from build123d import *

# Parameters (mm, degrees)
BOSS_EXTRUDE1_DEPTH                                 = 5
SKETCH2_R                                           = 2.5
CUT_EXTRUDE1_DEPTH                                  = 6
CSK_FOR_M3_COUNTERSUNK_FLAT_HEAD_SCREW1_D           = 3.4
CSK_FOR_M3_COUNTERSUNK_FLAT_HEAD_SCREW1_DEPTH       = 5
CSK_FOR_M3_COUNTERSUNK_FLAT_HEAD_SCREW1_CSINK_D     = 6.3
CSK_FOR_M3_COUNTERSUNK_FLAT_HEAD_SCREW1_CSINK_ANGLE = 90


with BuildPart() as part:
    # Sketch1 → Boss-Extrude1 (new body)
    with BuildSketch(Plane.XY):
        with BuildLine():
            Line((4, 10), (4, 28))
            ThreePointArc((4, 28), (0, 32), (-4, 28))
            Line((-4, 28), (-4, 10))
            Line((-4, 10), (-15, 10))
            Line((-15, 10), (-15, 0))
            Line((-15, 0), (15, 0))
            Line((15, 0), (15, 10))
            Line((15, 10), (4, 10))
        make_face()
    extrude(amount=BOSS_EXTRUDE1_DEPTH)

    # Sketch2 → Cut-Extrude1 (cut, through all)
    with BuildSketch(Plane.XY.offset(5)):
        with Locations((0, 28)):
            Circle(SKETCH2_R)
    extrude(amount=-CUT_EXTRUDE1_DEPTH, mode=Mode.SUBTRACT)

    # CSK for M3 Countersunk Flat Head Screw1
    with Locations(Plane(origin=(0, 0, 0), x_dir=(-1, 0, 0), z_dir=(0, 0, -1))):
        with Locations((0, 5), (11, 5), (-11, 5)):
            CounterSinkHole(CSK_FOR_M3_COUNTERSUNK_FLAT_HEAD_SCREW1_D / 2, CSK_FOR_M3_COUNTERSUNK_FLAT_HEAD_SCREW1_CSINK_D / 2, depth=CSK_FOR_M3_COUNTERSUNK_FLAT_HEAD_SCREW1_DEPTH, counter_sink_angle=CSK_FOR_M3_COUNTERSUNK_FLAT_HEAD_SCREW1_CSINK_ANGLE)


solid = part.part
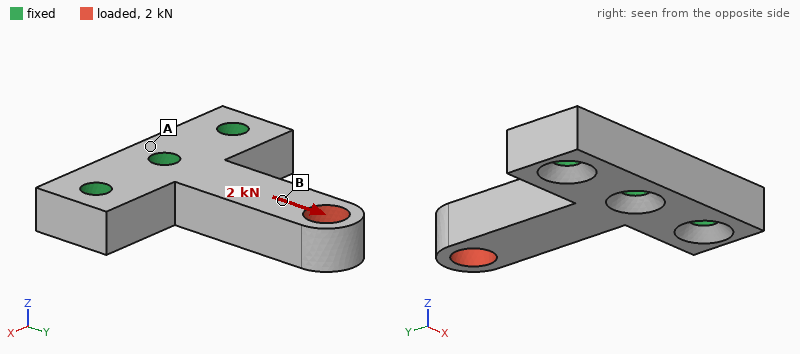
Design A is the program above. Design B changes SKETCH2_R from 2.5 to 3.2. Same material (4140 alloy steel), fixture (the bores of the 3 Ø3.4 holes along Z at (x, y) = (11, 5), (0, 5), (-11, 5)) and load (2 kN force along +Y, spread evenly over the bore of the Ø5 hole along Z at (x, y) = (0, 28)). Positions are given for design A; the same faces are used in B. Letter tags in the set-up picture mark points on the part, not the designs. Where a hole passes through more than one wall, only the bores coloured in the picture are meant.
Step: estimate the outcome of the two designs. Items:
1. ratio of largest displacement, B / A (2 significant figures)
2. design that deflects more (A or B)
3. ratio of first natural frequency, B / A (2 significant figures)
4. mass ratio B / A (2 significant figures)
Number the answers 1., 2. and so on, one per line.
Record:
1. 2.3
2. B
3. 1.1
4. 0.97
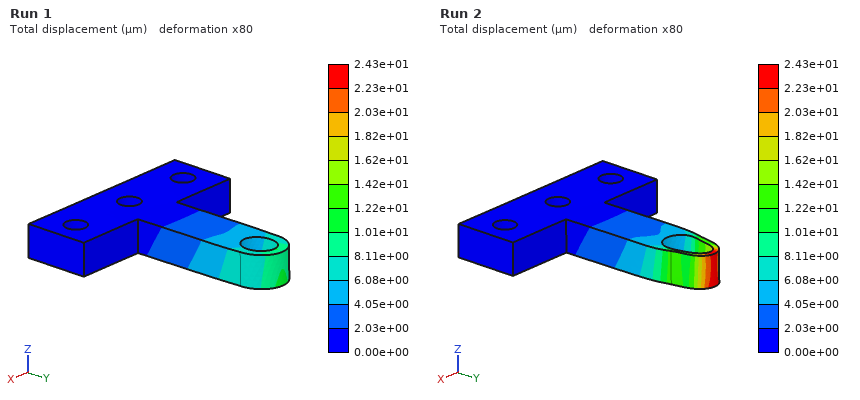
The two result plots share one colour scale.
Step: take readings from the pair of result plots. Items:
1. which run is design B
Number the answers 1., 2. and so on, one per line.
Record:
1. Run 2
